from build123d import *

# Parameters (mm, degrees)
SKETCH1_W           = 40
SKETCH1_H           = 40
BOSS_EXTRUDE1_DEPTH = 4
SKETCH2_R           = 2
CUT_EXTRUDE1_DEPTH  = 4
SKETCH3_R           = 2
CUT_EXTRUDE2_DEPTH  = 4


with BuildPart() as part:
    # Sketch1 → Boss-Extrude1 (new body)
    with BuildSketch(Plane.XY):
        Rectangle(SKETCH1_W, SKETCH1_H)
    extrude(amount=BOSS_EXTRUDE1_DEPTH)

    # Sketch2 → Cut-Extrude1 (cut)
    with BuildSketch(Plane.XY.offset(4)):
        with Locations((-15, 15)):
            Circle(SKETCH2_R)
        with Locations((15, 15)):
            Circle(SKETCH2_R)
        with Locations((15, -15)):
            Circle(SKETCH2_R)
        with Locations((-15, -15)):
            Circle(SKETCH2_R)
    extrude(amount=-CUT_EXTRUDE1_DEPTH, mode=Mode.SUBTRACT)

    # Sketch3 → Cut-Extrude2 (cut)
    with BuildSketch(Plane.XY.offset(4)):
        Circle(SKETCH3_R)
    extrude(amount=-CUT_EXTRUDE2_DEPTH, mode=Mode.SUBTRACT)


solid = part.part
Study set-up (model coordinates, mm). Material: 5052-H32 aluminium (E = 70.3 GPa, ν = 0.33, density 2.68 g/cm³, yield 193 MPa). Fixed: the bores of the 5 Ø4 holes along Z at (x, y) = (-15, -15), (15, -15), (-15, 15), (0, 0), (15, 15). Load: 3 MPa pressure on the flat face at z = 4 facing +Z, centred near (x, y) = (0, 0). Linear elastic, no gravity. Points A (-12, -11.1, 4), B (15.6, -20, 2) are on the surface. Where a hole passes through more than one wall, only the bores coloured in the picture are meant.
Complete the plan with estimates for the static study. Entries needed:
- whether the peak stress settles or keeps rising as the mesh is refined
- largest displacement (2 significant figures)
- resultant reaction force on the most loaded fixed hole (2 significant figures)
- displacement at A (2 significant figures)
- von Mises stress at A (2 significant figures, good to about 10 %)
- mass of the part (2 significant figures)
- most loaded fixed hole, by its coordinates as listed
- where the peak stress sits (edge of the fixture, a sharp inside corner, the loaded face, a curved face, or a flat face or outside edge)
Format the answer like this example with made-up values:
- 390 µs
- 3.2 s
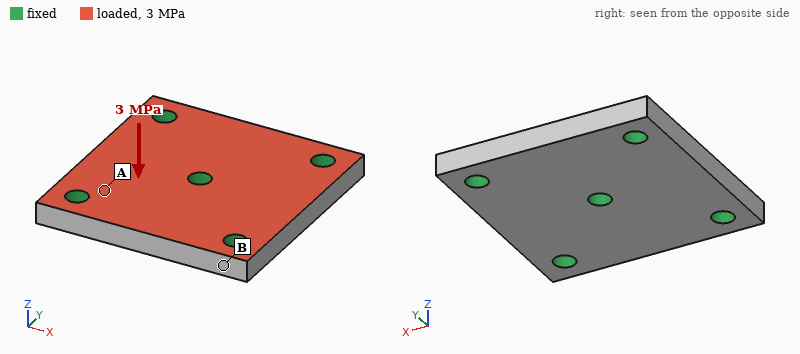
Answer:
- keeps rising
- 14 µm
- 1.3 kN
- 3.8 µm
- 28 MPa
- 16 g
- (0, 0)
- edge of the fixture
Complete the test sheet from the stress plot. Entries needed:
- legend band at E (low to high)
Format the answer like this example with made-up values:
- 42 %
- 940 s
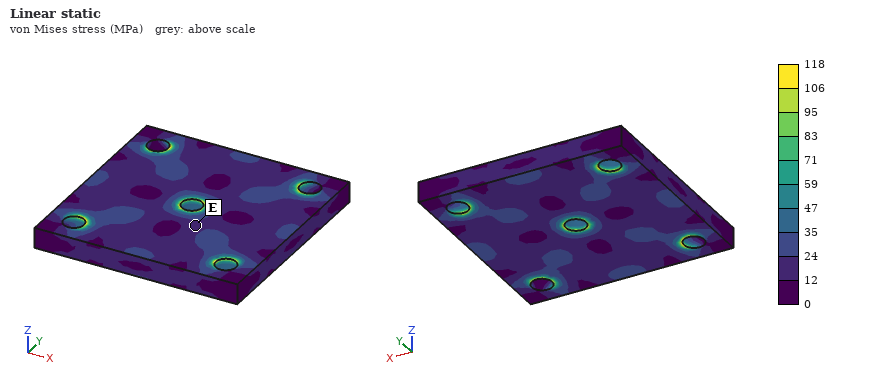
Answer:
- 12 to 24 MPa
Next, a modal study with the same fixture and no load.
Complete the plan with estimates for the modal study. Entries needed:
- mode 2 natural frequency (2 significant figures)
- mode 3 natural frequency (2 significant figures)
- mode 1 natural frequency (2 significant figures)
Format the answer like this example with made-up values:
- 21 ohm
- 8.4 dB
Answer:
- 27 kHz
- 27 kHz
- 26 kHz
